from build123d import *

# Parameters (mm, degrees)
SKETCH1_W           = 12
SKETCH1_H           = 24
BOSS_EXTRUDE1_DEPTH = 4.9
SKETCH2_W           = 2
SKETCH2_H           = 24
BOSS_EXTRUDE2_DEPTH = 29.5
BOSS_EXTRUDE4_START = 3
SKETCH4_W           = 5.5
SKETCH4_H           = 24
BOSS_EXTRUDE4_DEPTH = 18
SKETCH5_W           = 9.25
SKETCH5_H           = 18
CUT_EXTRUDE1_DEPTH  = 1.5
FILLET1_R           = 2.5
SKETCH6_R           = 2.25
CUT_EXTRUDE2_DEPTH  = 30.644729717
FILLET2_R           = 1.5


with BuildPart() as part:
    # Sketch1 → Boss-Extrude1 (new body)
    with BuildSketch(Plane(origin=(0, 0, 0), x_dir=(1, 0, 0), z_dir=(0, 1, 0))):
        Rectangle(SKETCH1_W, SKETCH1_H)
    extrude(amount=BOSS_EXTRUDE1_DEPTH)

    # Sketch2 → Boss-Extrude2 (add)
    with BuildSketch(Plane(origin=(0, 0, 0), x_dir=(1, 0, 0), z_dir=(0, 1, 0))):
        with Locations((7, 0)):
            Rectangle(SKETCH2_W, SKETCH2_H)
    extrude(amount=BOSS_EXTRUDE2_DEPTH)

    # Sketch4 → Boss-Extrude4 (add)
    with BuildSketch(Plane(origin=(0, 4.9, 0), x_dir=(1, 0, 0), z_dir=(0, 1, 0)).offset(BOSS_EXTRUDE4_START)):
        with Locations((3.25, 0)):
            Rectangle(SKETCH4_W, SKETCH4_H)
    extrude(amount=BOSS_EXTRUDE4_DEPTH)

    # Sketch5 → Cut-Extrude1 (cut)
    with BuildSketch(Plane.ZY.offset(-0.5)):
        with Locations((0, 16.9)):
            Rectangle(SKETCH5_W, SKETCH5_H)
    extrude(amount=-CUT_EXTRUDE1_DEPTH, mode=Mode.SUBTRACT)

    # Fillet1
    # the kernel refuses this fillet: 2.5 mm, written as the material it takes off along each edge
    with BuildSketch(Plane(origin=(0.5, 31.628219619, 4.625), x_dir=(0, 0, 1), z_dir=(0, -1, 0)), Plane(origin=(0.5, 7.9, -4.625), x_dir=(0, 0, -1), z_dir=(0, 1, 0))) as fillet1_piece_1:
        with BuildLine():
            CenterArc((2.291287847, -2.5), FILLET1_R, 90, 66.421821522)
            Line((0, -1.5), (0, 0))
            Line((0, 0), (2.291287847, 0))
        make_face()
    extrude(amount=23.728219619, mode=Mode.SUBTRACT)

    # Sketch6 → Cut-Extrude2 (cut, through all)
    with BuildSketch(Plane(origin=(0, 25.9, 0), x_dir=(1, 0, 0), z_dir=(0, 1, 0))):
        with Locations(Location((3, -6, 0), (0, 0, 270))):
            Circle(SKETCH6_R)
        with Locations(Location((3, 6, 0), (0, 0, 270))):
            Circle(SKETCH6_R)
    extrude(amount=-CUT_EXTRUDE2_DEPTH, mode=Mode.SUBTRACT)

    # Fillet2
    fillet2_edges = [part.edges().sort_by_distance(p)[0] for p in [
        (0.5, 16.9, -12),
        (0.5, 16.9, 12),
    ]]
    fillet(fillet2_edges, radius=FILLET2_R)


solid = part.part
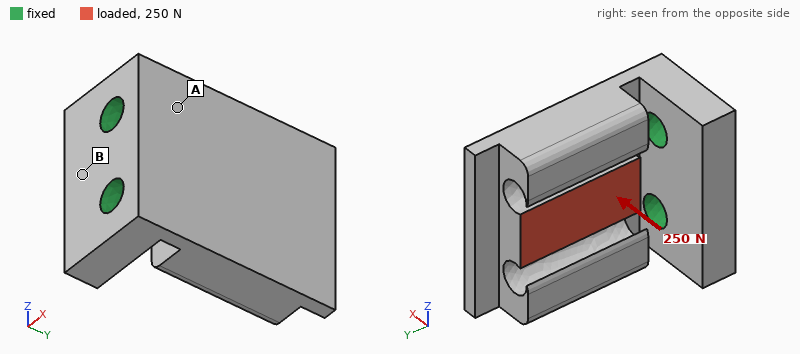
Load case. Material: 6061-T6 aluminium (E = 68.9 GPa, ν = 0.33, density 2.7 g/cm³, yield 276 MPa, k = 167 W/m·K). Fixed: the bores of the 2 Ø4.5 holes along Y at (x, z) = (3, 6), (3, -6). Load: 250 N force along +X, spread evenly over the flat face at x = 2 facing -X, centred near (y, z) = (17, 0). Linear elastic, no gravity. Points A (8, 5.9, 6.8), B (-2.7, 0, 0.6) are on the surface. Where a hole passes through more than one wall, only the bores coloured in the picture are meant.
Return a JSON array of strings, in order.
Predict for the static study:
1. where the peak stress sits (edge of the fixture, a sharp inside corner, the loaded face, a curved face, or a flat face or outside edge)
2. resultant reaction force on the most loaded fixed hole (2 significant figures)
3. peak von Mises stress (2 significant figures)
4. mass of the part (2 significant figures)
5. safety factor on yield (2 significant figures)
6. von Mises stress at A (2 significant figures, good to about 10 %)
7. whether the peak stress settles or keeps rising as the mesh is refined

["a flat face or outside edge", "130 N", "160 MPa", "11 g", "1.7", "150 MPa", "settles"]
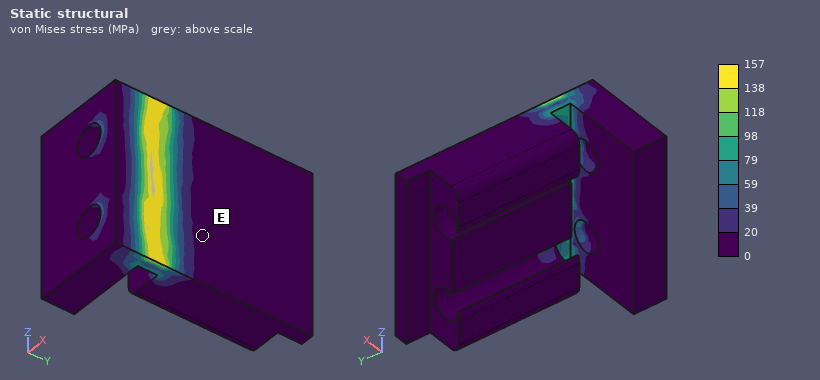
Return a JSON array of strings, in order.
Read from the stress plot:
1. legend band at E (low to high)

["0 to 20 MPa"]
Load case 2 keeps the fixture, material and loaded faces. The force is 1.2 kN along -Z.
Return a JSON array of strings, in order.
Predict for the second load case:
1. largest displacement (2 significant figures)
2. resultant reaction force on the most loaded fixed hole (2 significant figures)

["80 µm", "1.2 kN"]
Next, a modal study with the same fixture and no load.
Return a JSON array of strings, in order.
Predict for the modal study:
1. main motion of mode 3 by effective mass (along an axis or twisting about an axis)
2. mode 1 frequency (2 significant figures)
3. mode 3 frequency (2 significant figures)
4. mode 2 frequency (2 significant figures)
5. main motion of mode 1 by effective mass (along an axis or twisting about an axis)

["along Z", "2200 Hz", "11 kHz", "8500 Hz", "along X"]
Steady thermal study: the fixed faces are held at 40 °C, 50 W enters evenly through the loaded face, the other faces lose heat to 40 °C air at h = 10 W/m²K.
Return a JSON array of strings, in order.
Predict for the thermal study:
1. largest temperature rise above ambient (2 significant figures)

["69 K"]
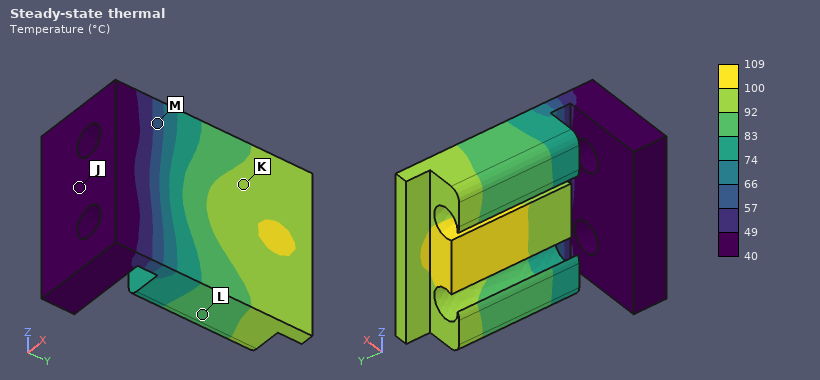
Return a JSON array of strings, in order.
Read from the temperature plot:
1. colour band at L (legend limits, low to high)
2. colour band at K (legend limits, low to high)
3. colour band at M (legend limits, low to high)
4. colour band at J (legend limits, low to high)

["83 to 92 °C", "92 to 100 °C", "57 to 66 °C", "40 to 49 °C"]
